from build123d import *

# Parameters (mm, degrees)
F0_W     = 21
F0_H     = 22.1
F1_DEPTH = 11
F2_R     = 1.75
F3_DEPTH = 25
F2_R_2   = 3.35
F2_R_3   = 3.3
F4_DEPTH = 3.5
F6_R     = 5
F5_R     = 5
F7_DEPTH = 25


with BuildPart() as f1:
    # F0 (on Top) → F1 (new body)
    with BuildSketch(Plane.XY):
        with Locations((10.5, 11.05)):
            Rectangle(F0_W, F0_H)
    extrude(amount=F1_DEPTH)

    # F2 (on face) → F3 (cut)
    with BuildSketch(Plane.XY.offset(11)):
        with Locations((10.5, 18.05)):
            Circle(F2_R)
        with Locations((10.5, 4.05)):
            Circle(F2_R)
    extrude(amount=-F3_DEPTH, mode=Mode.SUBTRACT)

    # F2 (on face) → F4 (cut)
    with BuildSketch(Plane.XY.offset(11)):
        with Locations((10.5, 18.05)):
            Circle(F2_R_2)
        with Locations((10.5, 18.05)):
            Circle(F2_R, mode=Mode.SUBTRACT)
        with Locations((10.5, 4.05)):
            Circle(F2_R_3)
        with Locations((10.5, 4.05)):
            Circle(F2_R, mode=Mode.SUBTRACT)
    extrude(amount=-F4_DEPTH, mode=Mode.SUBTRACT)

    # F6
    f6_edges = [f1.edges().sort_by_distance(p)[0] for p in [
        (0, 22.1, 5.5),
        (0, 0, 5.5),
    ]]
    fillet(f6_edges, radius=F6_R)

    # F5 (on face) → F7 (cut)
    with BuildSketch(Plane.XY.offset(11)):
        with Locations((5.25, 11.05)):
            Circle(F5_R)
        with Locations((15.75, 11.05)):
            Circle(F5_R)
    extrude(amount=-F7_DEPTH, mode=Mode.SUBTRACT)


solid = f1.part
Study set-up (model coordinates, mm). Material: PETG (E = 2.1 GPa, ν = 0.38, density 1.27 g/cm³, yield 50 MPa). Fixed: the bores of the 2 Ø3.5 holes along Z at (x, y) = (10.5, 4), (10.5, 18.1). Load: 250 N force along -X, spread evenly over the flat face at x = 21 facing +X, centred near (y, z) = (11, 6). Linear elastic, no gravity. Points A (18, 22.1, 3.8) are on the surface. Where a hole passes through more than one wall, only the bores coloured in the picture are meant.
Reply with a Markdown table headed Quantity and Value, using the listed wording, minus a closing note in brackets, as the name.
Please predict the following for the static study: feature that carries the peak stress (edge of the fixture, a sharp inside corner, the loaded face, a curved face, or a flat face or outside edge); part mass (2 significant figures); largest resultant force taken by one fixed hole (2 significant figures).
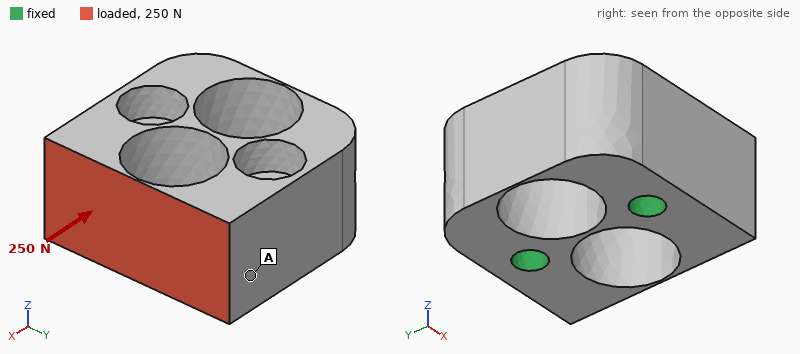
| Quantity | Value |
|---|---|
| feature that carries the peak stress | the loaded face |
| part mass | 3.6 g |
| largest resultant force taken by one fixed hole | 130 N |
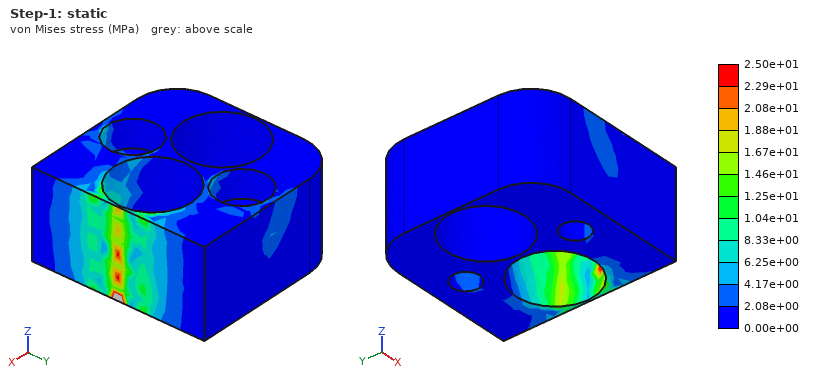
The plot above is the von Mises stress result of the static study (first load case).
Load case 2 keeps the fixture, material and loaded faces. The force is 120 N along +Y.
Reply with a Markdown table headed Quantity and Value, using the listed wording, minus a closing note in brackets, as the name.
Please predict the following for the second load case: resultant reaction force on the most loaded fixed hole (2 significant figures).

| Quantity | Value |
|---|---|
| resultant reaction force on the most loaded fixed hole | 61 N |
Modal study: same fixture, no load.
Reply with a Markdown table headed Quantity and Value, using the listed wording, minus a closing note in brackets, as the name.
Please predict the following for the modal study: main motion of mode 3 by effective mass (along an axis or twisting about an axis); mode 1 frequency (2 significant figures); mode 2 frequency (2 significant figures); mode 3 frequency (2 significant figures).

| Quantity | Value |
|---|---|
| main motion of mode 3 by effective mass | along Y |
| mode 1 frequency | 7600 Hz |
| mode 2 frequency | 8900 Hz |
| mode 3 frequency | 9800 Hz |
